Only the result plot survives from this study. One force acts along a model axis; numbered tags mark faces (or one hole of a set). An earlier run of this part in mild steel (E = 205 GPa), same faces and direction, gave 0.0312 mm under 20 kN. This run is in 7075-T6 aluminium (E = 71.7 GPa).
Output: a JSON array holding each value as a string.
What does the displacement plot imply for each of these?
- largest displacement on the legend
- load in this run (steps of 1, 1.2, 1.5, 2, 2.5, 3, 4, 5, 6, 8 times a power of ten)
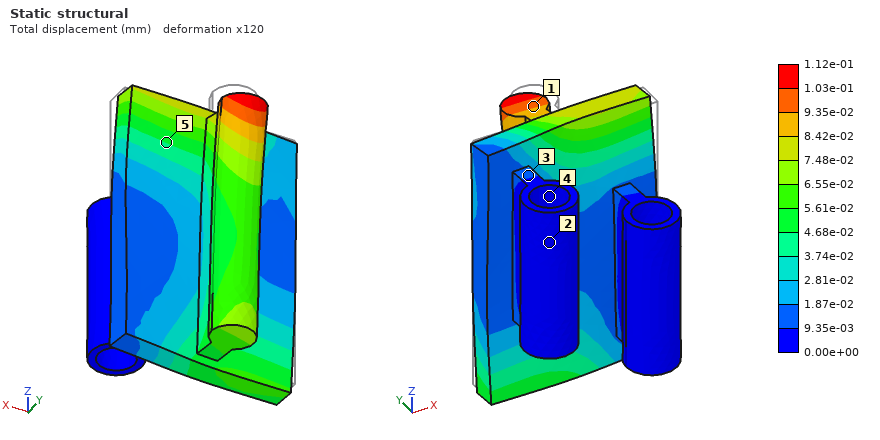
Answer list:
["1.12e-01 mm", "25 kN"]
